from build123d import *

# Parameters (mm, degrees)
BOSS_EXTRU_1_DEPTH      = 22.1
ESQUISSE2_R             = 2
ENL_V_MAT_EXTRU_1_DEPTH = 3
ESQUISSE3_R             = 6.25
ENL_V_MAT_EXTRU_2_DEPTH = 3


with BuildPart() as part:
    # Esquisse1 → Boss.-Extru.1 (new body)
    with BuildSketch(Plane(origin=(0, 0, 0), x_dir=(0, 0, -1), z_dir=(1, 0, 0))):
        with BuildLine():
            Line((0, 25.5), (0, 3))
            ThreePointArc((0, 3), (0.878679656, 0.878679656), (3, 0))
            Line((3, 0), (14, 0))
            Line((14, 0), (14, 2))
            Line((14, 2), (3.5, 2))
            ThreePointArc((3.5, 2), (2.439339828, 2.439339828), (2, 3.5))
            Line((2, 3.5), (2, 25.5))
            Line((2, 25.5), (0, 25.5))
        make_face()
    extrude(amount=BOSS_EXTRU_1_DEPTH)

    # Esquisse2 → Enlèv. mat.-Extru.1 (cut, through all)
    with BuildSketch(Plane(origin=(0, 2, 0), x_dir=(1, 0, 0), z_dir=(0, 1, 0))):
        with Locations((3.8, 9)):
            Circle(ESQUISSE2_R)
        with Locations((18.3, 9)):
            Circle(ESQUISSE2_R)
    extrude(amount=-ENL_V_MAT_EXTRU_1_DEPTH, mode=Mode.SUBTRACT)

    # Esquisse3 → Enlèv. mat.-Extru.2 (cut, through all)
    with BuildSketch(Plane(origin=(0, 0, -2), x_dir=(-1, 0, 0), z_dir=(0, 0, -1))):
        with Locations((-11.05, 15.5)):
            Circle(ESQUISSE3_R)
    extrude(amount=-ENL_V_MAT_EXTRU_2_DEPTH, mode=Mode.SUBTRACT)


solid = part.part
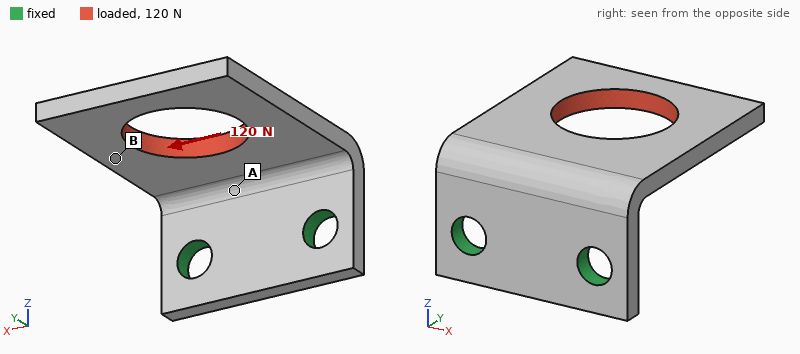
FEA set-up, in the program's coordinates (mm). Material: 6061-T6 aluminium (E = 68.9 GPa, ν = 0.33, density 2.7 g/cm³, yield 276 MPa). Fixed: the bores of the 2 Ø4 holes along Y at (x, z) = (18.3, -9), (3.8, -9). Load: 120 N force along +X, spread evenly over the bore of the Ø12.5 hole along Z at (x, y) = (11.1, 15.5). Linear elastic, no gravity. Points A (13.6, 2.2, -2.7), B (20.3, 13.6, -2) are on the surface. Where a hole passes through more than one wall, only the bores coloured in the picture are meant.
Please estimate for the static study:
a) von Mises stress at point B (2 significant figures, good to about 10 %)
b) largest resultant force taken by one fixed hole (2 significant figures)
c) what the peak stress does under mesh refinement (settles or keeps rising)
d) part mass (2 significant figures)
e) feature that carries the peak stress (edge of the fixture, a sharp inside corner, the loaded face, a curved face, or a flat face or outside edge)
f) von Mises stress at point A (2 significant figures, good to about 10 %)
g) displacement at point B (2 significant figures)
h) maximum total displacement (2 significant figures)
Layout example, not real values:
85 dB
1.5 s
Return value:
14 MPa
140 N
keeps rising
3.6 g
edge of the fixture
45 MPa
36 µm
62 µm
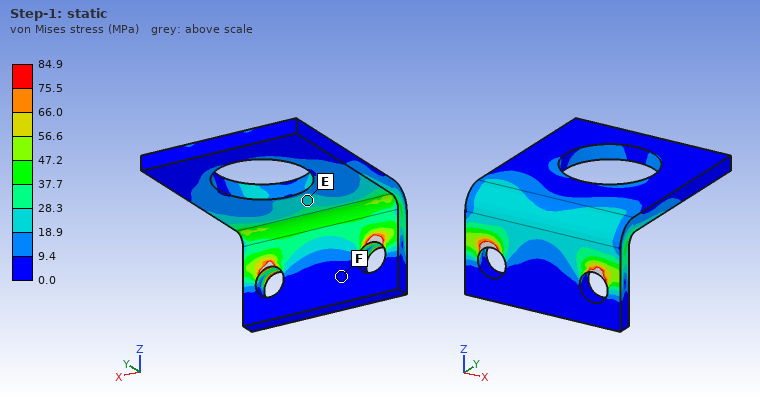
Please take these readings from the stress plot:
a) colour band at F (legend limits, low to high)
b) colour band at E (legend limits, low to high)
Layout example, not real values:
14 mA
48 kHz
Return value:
0.0 to 9.4 MPa
18.9 to 28.3 MPa
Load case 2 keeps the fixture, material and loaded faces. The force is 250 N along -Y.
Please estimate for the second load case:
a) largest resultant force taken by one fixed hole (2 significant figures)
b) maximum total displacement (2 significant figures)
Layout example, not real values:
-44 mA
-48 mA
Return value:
130 N
0.14 mm
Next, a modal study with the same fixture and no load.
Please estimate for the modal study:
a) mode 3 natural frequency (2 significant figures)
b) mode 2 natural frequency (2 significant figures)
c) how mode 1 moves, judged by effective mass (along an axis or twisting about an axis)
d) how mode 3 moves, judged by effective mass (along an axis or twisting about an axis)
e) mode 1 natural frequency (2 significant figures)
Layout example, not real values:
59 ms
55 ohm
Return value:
7200 Hz
5100 Hz
along Z
along X
2200 Hz
